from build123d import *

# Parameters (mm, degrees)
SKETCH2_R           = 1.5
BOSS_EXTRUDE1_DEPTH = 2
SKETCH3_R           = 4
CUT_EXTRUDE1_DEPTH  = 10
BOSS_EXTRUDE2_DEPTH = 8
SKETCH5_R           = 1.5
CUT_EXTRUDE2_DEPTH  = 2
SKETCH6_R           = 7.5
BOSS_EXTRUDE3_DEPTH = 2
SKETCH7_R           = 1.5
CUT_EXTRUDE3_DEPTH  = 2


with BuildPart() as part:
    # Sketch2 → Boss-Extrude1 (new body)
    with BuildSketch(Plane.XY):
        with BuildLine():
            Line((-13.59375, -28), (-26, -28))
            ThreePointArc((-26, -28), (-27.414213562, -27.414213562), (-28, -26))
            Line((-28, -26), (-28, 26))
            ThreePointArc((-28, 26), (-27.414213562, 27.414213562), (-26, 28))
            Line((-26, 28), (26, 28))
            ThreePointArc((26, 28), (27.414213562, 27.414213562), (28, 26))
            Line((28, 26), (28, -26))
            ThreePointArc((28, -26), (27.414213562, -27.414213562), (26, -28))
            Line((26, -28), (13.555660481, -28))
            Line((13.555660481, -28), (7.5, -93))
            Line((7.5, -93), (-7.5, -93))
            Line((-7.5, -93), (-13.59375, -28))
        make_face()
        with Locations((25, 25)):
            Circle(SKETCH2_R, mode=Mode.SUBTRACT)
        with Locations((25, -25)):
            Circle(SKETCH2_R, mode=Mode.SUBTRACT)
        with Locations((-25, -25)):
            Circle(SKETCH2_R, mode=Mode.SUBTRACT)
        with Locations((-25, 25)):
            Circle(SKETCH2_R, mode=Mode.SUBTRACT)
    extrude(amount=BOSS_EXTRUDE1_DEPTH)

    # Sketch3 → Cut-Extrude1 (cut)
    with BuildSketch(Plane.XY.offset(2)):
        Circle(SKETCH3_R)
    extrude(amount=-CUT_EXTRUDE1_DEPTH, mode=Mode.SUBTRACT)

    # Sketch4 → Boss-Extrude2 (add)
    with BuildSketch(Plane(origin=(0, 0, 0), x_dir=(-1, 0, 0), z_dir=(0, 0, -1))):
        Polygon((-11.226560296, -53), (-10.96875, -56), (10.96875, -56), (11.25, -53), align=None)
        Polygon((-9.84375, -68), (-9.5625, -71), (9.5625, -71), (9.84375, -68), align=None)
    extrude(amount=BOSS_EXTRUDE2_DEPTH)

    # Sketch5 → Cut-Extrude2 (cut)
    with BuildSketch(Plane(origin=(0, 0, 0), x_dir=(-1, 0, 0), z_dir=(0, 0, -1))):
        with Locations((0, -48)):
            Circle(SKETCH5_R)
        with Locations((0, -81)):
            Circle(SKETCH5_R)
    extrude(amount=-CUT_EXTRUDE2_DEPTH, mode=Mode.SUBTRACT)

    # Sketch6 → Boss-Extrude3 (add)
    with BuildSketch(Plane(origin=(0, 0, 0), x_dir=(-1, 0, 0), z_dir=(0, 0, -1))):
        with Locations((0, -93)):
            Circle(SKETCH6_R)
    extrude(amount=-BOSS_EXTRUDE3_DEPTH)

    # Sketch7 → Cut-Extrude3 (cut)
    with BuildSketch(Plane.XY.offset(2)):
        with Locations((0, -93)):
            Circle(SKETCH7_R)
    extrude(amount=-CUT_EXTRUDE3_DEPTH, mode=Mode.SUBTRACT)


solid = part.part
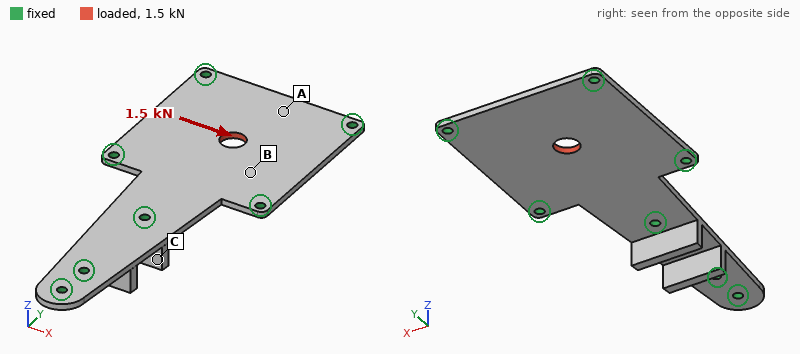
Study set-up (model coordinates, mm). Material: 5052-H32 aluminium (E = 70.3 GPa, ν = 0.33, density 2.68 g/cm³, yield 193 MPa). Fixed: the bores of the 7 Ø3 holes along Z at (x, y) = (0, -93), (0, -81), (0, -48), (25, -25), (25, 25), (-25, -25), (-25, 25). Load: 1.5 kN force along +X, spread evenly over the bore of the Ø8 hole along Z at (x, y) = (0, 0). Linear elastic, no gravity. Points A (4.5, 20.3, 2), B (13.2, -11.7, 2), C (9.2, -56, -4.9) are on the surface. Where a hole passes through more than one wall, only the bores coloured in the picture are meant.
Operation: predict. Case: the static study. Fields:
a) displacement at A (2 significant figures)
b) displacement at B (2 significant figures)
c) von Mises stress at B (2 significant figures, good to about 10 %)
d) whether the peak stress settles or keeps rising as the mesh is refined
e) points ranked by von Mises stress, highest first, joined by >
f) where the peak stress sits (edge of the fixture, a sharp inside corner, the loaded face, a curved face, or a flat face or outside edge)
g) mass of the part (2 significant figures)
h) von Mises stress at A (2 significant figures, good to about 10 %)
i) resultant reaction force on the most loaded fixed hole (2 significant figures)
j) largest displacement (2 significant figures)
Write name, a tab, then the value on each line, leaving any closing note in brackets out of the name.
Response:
displacement at A	4.0 µm
displacement at B	5.8 µm
von Mises stress at B	15 MPa
whether the peak stress settles or keeps rising as the mesh is refined	keeps rising
points ranked by von Mises stress, highest first, joined by >	B > A > C
where the peak stress sits	edge of the fixture
mass of the part	27 g
von Mises stress at A	8.1 MPa
resultant reaction force on the most loaded fixed hole	420 N
largest displacement	11 µm
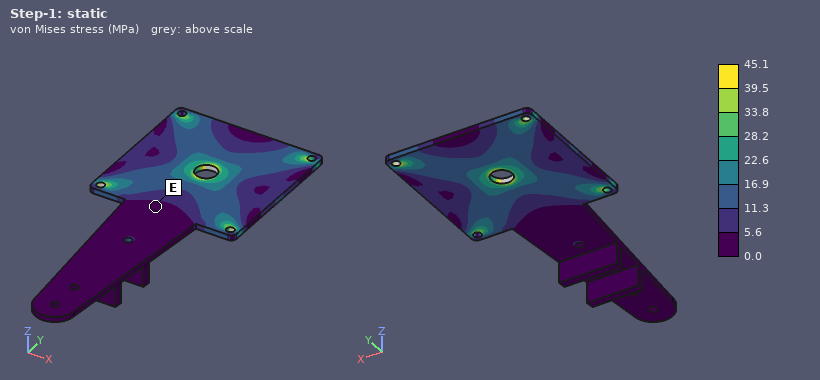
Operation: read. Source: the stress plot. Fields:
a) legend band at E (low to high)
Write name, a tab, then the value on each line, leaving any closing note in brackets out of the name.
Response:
legend band at E	0.0 to 5.6 MPa
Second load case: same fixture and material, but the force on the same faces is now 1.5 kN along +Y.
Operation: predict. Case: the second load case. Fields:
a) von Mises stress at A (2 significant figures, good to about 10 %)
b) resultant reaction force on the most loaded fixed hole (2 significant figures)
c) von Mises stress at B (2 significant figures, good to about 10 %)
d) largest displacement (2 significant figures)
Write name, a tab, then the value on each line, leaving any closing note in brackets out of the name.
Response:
von Mises stress at A	5.8 MPa
resultant reaction force on the most loaded fixed hole	330 N
von Mises stress at B	12 MPa
largest displacement	9.6 µm
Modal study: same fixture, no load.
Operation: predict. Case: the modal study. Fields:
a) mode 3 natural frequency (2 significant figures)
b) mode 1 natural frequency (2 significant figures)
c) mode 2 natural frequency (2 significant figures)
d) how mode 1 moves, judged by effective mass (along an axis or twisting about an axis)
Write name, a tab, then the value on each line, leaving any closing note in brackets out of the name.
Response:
mode 3 natural frequency	4900 Hz
mode 1 natural frequency	2700 Hz
mode 2 natural frequency	4800 Hz
how mode 1 moves, judged by effective mass	along Z
